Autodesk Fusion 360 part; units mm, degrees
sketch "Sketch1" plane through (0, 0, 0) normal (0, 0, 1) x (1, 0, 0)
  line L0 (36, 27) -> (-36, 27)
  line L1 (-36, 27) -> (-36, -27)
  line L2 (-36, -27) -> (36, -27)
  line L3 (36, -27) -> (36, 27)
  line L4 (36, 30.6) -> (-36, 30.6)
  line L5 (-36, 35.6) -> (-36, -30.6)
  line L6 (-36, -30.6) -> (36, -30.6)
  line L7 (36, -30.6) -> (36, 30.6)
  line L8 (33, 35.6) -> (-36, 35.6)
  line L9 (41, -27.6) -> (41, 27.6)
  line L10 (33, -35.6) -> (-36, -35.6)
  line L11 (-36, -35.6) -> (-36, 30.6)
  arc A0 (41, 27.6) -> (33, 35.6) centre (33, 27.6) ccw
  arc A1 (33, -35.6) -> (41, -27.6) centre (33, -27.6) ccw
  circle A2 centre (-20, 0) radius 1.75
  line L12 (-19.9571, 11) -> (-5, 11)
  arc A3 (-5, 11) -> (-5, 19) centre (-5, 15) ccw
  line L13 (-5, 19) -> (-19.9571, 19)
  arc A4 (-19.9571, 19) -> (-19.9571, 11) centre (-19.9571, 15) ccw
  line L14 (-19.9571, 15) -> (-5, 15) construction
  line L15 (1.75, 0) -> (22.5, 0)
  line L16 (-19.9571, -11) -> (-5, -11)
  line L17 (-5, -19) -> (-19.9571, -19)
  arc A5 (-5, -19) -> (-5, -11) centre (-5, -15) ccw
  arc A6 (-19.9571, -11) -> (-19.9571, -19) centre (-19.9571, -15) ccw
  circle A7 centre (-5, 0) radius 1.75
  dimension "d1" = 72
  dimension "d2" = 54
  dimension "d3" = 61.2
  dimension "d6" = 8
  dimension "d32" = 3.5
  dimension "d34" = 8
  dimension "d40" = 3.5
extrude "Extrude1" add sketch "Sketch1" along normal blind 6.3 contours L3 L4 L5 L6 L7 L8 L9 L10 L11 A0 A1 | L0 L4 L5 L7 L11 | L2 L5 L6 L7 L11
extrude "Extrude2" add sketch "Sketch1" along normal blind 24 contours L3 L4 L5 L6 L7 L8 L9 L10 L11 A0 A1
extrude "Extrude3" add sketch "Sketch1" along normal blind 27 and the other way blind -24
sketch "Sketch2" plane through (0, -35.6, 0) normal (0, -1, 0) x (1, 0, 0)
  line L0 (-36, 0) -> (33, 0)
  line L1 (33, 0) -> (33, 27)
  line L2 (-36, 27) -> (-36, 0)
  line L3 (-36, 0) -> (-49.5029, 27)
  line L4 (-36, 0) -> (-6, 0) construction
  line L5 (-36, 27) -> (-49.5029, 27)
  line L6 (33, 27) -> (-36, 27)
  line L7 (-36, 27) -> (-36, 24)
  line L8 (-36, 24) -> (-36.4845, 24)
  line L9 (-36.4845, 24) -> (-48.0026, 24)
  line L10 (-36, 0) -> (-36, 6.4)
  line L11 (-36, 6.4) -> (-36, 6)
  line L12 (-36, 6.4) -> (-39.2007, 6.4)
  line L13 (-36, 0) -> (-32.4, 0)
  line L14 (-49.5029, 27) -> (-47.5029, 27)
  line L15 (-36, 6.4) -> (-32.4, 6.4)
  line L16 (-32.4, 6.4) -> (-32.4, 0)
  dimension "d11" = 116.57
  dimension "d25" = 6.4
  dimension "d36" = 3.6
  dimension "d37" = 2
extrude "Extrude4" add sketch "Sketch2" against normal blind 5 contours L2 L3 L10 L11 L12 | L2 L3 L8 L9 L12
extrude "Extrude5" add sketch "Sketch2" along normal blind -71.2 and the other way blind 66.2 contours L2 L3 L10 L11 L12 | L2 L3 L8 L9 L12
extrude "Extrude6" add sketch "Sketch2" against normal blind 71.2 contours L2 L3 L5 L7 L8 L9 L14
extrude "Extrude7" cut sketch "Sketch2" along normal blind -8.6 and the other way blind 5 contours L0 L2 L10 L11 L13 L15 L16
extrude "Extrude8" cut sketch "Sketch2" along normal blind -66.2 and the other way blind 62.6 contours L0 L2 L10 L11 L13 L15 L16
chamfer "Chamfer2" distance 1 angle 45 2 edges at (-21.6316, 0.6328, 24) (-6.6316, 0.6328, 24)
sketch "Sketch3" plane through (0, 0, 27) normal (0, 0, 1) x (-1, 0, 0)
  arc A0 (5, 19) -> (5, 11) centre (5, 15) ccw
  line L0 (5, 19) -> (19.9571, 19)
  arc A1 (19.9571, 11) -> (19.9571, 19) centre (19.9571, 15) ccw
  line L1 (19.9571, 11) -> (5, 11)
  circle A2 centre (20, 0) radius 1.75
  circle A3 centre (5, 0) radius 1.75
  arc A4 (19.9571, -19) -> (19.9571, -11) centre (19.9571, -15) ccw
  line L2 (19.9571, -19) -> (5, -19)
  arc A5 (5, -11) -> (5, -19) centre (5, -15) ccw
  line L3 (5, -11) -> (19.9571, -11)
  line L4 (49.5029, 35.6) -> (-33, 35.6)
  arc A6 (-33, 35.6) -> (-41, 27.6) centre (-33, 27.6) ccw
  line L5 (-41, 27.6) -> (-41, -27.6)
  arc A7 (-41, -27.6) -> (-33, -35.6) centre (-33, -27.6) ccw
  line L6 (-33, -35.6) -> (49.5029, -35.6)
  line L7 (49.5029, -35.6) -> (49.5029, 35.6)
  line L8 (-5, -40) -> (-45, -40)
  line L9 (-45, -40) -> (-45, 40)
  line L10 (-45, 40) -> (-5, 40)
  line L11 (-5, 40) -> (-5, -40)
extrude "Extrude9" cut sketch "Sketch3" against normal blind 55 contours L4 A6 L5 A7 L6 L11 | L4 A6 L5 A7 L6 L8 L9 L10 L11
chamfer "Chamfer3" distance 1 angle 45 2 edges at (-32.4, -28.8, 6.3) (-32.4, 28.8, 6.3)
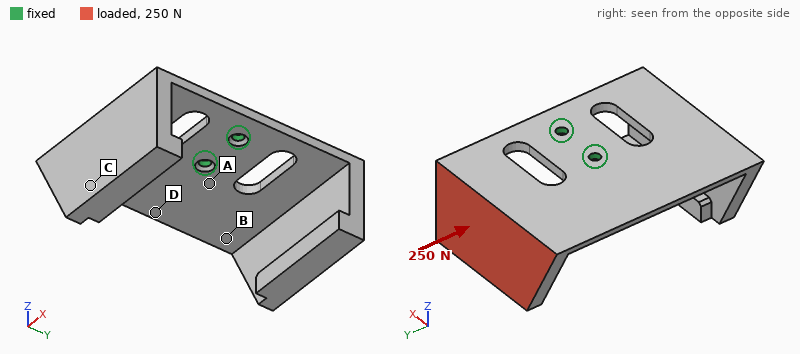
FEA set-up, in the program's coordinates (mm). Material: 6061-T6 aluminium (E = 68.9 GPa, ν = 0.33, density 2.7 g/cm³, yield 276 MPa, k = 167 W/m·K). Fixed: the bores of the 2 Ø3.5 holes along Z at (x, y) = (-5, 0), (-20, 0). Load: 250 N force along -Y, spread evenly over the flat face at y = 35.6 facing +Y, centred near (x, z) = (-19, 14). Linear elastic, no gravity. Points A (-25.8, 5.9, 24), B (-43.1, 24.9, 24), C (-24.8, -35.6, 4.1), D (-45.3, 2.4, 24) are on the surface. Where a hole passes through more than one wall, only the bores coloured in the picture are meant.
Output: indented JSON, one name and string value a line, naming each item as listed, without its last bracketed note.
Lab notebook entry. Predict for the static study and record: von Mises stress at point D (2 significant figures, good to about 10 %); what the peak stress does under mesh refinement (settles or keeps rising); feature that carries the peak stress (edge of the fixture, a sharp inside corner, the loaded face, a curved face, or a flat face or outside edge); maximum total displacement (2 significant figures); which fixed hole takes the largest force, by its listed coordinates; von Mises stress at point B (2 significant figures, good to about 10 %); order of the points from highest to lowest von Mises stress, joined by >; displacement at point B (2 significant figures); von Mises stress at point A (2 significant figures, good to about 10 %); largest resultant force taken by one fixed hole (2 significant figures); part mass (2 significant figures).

{
  "von Mises stress at point D": "30 MPa",
  "what the peak stress does under mesh refinement": "keeps rising",
  "feature that carries the peak stress": "edge of the fixture",
  "maximum total displacement": "0.60 mm",
  "which fixed hole takes the largest force, by its listed coordinates": "(-20, 0)",
  "von Mises stress at point B": "41 MPa",
  "order of the points from highest to lowest von Mises stress, joined by >": "A > B > D > C",
  "displacement at point B": "0.23 mm",
  "von Mises stress at point A": "54 MPa",
  "largest resultant force taken by one fixed hole": "210 N",
  "part mass": "63 g"
}
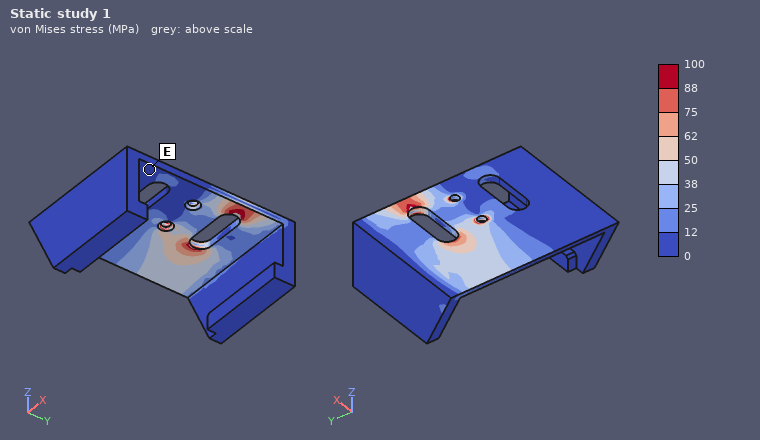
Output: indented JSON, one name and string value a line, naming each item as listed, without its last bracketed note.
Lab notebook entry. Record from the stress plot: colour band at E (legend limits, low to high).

{
  "colour band at E": "0 to 12 MPa"
}
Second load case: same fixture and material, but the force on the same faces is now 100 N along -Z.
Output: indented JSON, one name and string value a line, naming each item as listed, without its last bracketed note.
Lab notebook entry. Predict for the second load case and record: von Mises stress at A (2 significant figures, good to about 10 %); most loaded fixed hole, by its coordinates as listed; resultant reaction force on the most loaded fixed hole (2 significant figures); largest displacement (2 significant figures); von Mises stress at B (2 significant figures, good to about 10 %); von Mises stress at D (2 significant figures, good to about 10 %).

{
  "von Mises stress at A": "50 MPa",
  "most loaded fixed hole, by its coordinates as listed": "(-20, 0)",
  "resultant reaction force on the most loaded fixed hole": "79 N",
  "largest displacement": "0.50 mm",
  "von Mises stress at B": "19 MPa",
  "von Mises stress at D": "26 MPa"
}
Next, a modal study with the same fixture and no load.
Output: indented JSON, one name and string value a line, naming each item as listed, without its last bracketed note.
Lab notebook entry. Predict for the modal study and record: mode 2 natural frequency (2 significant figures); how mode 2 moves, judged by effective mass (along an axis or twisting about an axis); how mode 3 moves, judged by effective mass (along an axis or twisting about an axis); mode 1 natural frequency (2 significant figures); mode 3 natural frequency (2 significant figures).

{
  "mode 2 natural frequency": "640 Hz",
  "how mode 2 moves, judged by effective mass": "along Z",
  "how mode 3 moves, judged by effective mass": "along X",
  "mode 1 natural frequency": "480 Hz",
  "mode 3 natural frequency": "1100 Hz"
}
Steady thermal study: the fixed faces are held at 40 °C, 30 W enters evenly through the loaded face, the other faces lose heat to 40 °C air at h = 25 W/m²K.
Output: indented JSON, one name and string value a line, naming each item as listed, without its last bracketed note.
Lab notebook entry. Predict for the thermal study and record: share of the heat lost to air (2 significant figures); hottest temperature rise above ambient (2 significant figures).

{
  "share of the heat lost to air": "23 %",
  "hottest temperature rise above ambient": "61 K"
}
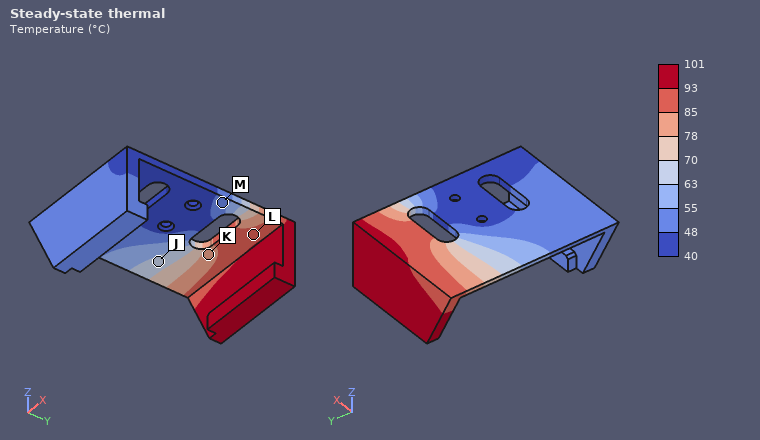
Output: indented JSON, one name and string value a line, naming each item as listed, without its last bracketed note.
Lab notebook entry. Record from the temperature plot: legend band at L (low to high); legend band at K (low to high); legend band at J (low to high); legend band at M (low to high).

{
  "legend band at L": "85 to 93 °C",
  "legend band at K": "78 to 85 °C",
  "legend band at J": "63 to 70 °C",
  "legend band at M": "48 to 55 °C"
}
